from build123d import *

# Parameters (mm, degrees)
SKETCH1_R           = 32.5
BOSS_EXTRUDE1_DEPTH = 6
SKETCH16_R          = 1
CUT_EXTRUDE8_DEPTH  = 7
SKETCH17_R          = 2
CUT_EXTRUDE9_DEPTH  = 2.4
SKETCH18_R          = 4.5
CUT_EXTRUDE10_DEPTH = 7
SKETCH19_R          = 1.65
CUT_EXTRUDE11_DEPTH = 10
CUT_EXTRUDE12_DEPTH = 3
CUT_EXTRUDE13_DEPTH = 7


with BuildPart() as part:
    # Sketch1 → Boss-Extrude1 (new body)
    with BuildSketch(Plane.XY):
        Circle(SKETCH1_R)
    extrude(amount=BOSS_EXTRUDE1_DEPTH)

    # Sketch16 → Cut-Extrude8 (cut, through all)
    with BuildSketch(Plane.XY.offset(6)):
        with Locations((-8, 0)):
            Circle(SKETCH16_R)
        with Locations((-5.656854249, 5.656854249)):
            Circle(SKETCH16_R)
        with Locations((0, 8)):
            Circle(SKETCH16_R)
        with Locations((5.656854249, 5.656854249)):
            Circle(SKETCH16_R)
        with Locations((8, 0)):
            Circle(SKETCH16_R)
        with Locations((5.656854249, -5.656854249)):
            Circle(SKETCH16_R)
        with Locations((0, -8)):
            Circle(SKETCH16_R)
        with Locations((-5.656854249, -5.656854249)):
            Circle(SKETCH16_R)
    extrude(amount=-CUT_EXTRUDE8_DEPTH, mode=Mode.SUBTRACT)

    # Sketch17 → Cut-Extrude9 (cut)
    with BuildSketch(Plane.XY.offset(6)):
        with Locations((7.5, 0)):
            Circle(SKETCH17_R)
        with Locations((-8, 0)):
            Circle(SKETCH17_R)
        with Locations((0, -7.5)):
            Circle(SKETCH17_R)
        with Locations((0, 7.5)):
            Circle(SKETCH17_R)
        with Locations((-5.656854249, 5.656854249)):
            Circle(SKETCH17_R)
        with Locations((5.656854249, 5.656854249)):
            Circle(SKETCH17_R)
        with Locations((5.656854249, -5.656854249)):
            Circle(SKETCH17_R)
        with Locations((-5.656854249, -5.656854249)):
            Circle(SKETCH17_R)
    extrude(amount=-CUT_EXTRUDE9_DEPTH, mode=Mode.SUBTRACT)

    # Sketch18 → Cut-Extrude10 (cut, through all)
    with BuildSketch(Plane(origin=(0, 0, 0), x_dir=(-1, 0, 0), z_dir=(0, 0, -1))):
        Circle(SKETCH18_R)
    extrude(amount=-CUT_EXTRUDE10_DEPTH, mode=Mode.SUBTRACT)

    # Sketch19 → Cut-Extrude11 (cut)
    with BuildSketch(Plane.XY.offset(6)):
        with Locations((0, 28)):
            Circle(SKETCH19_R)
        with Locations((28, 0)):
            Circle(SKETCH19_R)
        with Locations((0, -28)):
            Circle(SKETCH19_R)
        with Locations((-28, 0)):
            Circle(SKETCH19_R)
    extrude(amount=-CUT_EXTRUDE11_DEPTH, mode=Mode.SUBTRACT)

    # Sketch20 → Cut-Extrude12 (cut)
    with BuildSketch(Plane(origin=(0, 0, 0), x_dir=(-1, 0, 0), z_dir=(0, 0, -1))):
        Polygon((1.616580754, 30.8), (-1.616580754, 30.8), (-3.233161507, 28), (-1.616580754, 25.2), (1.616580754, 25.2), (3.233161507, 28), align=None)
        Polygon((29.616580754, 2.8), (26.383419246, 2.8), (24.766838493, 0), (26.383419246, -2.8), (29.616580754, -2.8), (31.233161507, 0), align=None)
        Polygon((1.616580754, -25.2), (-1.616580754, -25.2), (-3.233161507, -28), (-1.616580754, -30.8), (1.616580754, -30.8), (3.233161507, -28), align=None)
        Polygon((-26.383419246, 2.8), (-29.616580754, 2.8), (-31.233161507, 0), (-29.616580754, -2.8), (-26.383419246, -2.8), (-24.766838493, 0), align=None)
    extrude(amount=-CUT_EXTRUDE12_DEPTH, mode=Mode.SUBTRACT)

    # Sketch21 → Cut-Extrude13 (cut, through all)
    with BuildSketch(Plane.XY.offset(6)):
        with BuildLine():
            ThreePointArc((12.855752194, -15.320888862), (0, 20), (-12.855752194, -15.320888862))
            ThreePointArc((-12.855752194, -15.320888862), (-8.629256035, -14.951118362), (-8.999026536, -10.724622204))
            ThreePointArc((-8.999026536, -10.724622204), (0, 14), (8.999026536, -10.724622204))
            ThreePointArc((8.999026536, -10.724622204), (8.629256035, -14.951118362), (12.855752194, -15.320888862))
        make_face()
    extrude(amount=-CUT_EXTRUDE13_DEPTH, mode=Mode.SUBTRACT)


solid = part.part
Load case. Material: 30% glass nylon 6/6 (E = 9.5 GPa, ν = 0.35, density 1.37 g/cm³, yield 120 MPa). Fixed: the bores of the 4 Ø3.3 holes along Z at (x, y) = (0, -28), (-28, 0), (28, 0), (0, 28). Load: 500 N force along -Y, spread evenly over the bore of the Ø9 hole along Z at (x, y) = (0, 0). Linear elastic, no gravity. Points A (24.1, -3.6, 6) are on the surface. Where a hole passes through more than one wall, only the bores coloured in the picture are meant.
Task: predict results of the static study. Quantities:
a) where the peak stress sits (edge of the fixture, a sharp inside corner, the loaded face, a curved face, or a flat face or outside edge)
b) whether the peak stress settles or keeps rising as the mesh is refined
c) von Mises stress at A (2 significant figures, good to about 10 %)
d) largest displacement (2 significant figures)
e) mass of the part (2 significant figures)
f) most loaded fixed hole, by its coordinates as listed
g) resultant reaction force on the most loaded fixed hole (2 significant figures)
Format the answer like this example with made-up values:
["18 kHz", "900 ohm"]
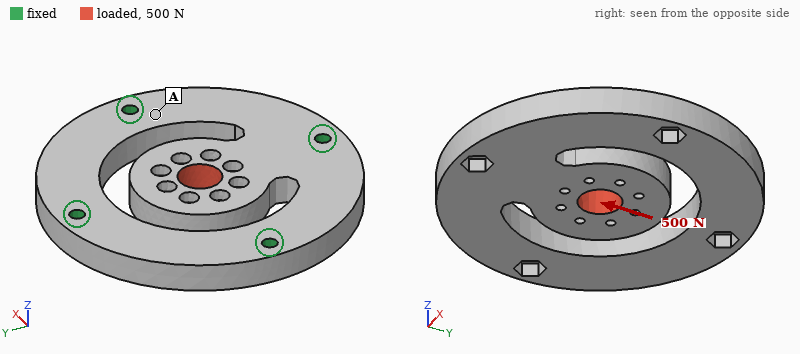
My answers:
["edge of the fixture", "keeps rising", "2.6 MPa", "38 µm", "21 g", "(0, -28)", "370 N"]
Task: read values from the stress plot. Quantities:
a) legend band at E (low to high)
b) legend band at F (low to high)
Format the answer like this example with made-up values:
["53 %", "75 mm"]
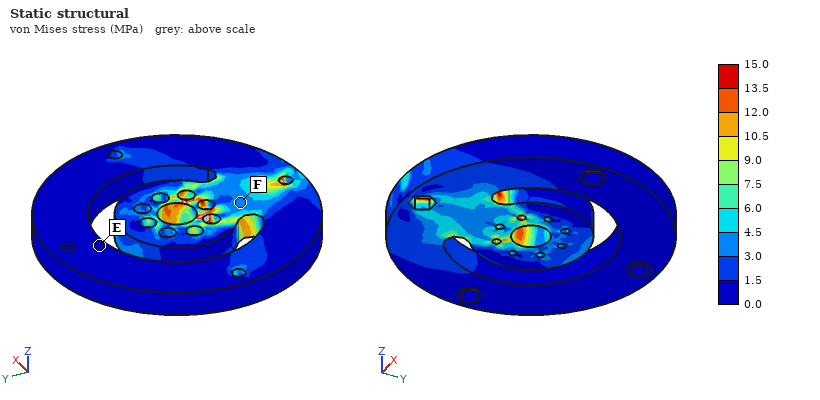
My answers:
["0.0 to 1.5 MPa", "3.0 to 4.5 MPa"]
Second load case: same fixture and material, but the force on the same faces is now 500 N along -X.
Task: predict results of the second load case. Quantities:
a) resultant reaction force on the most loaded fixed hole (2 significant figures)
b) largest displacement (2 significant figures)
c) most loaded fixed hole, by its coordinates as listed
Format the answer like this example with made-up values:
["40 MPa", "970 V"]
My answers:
["530 N", "0.31 mm", "(0, -28)"]
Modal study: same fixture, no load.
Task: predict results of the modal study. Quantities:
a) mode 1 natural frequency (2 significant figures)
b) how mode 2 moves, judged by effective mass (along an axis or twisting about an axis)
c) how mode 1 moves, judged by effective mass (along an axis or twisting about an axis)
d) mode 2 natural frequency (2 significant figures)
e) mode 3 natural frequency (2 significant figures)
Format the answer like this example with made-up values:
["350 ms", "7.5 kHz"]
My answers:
["1400 Hz", "along X", "along Z", "3500 Hz", "4000 Hz"]
